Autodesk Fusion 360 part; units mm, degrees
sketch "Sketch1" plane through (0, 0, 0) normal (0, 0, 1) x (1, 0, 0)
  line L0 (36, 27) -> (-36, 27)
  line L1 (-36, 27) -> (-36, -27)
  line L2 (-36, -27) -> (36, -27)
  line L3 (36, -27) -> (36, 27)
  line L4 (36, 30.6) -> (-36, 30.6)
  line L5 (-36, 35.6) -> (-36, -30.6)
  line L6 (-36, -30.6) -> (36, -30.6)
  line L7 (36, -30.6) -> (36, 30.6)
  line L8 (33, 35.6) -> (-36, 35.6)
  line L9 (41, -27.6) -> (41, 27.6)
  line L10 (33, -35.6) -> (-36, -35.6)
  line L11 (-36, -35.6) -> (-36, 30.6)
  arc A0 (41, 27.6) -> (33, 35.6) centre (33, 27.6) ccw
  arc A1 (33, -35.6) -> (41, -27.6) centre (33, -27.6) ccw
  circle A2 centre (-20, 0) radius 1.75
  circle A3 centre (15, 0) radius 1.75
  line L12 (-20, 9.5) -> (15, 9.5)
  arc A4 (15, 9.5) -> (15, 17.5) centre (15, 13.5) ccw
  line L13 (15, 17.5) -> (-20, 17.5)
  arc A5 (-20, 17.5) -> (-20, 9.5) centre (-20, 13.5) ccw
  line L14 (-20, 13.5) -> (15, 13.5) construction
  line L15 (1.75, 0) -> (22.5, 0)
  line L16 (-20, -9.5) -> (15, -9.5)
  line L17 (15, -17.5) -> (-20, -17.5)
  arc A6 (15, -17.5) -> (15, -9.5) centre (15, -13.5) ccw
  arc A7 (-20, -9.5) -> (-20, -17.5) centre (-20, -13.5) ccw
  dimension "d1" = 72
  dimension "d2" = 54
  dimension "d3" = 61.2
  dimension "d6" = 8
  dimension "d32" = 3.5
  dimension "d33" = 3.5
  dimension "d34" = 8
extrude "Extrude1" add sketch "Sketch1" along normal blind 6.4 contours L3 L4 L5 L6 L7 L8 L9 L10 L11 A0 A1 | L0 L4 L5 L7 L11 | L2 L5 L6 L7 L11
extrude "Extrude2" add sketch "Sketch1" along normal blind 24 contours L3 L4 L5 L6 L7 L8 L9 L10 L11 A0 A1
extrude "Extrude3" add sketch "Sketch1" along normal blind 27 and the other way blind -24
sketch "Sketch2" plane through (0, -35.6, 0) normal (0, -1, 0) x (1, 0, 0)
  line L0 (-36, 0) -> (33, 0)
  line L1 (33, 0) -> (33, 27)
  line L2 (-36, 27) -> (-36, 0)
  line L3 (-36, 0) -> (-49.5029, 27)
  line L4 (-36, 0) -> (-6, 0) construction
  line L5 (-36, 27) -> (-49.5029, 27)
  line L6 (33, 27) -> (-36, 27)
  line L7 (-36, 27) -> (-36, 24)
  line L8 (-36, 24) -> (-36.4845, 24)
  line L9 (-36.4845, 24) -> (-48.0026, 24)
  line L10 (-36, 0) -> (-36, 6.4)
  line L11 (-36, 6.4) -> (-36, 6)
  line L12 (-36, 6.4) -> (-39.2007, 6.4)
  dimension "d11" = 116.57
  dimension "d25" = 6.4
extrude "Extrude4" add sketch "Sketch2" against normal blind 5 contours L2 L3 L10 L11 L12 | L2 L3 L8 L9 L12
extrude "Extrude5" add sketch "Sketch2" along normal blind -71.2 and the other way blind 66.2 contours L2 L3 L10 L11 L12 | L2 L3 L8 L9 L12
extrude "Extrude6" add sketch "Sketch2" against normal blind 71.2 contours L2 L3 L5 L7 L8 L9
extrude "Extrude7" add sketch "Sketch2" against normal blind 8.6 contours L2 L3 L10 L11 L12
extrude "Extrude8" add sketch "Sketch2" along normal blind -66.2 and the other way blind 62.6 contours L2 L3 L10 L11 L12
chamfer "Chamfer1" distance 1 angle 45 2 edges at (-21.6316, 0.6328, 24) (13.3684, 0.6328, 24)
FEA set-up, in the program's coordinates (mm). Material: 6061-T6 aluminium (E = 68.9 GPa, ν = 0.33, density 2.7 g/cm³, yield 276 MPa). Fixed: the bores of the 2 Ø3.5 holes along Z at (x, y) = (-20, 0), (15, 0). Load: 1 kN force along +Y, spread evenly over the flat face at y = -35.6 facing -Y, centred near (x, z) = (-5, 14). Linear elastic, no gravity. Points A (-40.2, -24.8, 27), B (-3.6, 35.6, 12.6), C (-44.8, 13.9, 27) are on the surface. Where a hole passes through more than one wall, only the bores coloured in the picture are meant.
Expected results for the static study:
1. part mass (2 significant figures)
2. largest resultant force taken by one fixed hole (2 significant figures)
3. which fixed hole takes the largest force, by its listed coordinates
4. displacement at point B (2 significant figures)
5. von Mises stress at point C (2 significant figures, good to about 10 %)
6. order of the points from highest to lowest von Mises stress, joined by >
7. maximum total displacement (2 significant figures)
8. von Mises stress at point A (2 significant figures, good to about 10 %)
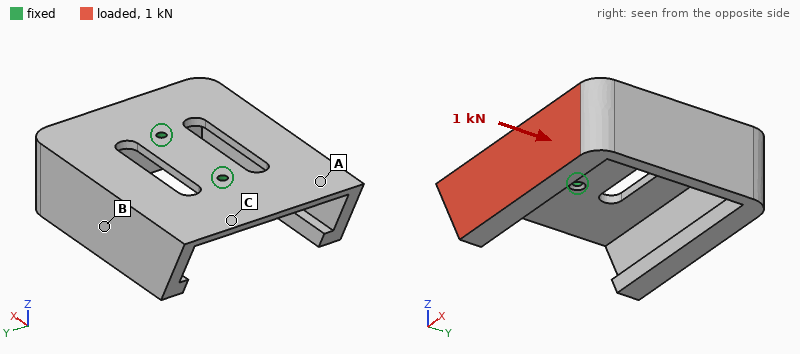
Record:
130 g
580 N
(-20, 0)
0.63 mm
33 MPa
A > C > B
0.95 mm
56 MPa
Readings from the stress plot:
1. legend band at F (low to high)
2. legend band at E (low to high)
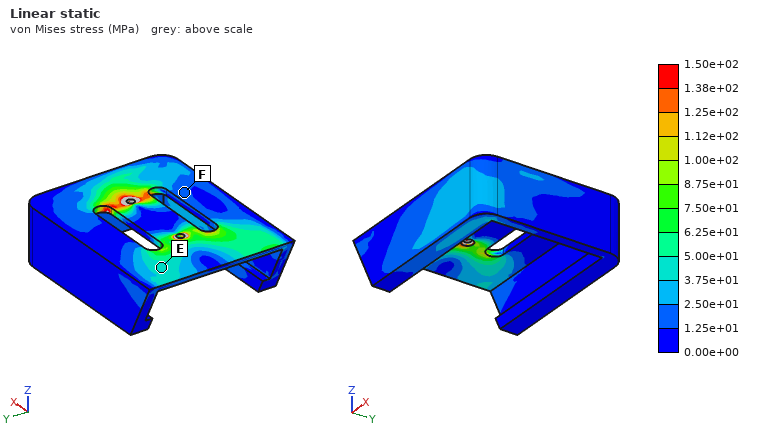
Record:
1.25e+01 to 2.50e+01 MPa
3.75e+01 to 5.00e+01 MPa
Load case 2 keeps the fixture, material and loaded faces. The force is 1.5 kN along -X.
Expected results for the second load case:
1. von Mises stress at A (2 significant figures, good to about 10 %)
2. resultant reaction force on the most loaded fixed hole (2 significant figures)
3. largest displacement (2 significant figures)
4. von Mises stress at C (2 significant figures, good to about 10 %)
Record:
34 MPa
1.6 kN
0.37 mm
42 MPa
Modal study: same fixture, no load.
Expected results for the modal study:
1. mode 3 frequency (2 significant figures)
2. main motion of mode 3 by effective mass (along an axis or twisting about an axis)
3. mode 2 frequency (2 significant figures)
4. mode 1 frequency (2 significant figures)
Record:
1200 Hz
along Z
940 Hz
400 Hz
